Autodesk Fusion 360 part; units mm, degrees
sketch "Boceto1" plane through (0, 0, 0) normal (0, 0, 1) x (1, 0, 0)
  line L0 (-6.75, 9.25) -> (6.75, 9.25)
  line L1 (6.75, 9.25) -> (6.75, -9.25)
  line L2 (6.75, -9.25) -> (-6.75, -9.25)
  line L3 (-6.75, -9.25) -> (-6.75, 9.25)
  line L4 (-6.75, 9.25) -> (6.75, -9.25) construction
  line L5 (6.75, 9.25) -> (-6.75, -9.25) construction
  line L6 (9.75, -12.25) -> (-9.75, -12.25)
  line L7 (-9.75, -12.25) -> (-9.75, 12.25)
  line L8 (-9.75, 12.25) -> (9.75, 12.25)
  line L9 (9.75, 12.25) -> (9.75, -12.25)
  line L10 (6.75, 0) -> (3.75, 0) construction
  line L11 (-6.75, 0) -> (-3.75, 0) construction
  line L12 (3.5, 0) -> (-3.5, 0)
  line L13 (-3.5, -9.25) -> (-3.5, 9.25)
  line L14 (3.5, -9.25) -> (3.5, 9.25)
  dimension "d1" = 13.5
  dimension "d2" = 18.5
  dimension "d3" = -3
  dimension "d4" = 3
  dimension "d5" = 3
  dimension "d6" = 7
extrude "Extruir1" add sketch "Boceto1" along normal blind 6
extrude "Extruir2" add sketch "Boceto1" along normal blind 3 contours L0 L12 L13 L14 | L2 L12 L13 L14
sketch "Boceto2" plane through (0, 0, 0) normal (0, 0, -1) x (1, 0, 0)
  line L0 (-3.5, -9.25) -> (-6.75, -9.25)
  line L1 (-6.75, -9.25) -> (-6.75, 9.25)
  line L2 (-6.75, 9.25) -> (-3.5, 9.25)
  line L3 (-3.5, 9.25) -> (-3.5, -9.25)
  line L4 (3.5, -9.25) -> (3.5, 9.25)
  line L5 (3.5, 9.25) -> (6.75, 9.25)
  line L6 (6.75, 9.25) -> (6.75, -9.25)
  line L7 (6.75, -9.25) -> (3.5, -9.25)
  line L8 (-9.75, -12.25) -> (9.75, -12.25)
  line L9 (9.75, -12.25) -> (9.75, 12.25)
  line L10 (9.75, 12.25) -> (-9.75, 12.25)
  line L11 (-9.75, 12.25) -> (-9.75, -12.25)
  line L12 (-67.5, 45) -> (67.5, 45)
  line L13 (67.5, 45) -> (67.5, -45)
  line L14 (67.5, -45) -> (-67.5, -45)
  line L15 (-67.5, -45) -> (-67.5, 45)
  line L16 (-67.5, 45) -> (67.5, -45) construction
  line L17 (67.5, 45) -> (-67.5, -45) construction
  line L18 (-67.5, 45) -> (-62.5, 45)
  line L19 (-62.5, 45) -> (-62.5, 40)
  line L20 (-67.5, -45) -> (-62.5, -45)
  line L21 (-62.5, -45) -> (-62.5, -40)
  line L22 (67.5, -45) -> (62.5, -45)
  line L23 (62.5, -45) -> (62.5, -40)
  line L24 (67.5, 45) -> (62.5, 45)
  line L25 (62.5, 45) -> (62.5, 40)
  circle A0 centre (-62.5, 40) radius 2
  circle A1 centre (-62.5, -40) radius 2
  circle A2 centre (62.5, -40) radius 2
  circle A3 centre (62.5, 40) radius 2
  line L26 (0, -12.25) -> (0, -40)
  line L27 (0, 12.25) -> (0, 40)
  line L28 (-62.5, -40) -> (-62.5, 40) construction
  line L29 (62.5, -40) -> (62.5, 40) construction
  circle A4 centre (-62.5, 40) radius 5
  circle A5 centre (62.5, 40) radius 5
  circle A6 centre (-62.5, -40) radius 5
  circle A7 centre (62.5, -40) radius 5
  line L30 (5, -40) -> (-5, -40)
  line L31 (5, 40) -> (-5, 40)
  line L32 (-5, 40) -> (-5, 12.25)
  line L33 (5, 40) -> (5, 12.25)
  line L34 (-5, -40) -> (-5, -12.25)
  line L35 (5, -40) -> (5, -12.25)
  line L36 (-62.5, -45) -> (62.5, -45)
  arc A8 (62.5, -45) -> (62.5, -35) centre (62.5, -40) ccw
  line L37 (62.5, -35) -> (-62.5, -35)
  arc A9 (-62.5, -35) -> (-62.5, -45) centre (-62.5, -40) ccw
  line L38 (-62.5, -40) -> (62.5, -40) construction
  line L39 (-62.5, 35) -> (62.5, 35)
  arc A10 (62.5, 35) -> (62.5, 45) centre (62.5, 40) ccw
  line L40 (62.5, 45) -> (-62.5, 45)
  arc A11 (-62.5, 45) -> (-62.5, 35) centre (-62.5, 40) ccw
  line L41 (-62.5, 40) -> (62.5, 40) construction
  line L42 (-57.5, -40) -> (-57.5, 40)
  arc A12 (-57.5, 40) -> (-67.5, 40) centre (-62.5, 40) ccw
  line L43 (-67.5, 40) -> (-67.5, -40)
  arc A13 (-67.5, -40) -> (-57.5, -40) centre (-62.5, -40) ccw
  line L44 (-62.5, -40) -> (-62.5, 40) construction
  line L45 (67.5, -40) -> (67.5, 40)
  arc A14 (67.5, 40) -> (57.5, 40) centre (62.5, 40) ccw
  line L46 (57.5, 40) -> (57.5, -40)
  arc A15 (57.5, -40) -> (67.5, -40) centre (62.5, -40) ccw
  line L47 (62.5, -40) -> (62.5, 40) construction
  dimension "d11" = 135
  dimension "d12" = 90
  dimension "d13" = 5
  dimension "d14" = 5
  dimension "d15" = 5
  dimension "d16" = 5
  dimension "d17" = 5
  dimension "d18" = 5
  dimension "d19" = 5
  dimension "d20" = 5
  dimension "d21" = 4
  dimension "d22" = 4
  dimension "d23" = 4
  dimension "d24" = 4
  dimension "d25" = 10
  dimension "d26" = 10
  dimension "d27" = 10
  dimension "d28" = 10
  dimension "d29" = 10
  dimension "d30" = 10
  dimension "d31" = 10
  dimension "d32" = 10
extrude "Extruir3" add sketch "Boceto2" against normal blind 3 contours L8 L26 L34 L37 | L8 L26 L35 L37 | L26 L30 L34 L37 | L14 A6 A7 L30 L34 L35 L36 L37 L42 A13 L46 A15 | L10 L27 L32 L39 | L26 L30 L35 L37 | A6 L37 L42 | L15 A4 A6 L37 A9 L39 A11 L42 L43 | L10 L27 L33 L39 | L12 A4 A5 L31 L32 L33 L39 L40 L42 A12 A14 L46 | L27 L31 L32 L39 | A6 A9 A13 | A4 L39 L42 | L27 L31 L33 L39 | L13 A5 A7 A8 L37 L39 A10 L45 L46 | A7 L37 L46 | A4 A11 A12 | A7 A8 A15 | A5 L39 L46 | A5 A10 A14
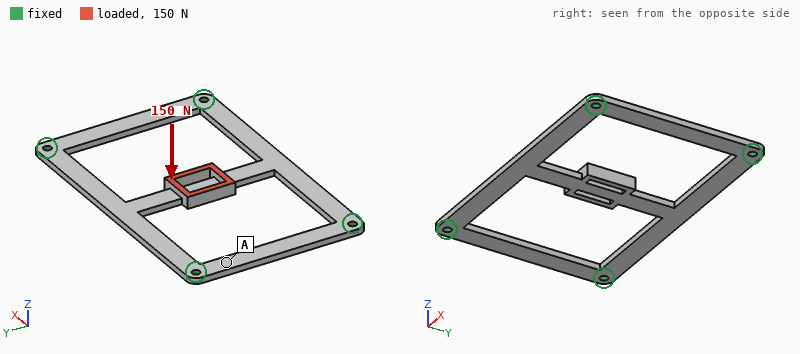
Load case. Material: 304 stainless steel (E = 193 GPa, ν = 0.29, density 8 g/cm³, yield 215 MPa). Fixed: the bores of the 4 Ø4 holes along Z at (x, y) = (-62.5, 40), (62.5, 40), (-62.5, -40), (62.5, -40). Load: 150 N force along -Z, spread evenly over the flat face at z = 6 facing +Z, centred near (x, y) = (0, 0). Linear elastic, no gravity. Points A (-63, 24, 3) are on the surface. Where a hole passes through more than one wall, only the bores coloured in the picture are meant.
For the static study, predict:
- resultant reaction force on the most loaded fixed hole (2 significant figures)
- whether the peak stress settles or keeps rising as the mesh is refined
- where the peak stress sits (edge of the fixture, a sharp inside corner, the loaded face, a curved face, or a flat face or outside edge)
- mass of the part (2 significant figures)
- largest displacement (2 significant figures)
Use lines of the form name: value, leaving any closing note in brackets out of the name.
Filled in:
resultant reaction force on the most loaded fixed hole: 38 N
whether the peak stress settles or keeps rising as the mesh is refined: keeps rising
where the peak stress sits: edge of the fixture
mass of the part: 120 g
largest displacement: 0.27 mm
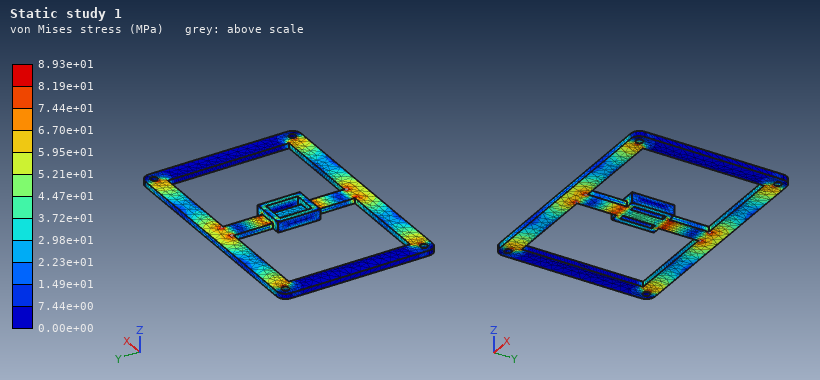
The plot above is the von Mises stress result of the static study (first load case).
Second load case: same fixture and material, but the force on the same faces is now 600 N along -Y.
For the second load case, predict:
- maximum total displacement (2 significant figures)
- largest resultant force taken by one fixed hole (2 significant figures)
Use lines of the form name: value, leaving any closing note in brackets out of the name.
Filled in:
maximum total displacement: 96 µm
largest resultant force taken by one fixed hole: 150 N
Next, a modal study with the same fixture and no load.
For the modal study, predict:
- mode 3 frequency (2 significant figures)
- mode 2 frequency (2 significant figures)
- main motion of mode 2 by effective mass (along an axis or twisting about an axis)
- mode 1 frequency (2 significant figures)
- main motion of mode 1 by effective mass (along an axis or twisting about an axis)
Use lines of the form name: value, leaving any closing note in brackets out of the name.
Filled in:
mode 3 frequency: 2000 Hz
mode 2 frequency: 990 Hz
main motion of mode 2 by effective mass: twisting about X
mode 1 frequency: 660 Hz
main motion of mode 1 by effective mass: along Z
